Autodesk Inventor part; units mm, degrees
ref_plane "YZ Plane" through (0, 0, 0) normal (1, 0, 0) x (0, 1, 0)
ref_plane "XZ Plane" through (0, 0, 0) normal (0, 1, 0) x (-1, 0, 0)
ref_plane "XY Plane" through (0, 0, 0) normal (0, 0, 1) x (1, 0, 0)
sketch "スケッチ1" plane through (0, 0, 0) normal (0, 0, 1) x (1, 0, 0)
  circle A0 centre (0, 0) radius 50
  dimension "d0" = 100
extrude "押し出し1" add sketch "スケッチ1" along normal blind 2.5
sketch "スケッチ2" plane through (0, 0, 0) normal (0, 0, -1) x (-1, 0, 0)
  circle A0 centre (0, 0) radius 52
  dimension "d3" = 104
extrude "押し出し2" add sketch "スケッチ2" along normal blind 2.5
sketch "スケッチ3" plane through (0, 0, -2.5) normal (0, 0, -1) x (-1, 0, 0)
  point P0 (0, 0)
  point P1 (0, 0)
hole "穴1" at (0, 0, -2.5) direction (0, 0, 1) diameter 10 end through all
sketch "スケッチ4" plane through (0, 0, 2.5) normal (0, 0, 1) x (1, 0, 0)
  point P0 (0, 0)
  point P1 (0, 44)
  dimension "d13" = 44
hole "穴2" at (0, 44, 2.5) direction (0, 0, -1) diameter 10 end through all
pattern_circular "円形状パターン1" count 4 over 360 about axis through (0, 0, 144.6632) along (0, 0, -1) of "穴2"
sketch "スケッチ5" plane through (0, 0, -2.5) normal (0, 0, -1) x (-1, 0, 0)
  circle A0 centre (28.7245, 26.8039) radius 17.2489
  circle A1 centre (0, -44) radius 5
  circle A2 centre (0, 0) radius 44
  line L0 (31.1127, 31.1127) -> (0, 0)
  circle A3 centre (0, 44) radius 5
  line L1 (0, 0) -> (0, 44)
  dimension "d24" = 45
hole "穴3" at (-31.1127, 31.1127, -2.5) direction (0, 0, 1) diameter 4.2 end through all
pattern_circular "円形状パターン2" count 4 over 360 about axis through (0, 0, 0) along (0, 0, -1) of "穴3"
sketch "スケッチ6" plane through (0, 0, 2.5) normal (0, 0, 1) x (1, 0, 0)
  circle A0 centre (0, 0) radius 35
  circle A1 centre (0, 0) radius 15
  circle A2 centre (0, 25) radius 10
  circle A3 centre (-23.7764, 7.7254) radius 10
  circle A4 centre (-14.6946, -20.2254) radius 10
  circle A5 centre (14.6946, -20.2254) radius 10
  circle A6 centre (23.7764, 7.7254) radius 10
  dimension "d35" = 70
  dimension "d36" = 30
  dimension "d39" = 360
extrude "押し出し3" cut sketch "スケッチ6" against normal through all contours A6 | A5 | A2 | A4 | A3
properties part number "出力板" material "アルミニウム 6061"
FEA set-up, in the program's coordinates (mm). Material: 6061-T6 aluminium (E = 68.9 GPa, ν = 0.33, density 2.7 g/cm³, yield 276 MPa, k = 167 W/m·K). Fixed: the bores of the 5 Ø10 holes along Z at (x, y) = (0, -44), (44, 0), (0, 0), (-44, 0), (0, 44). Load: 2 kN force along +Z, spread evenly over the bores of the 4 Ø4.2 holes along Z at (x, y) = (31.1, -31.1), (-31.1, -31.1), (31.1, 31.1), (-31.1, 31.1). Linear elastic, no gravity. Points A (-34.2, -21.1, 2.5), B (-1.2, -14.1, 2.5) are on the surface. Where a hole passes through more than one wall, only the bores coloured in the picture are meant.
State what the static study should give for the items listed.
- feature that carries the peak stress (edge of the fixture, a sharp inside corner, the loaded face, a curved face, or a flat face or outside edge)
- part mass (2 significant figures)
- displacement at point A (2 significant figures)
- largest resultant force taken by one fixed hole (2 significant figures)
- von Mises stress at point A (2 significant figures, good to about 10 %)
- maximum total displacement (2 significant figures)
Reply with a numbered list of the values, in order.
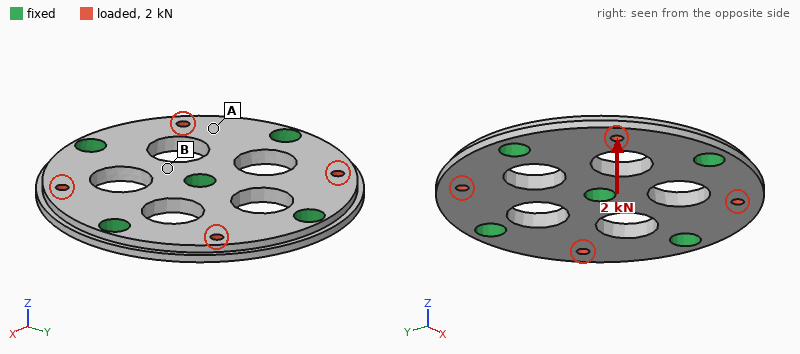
1. the loaded face
2. 83 g
3. 34 µm
4. 510 N
5. 20 MPa
6. 80 µm
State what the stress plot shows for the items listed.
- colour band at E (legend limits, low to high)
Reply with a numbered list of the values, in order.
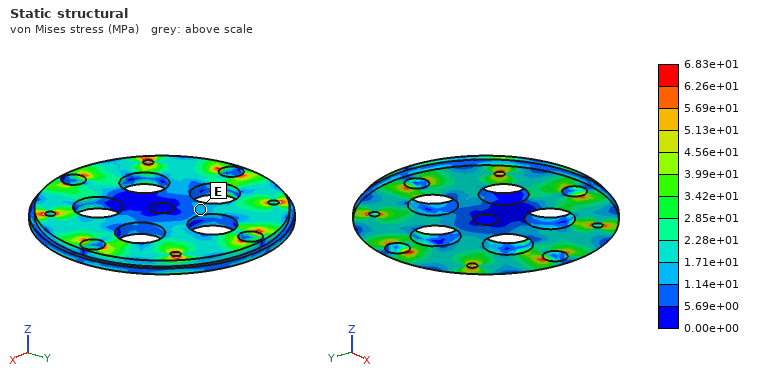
1. 1.14e+01 to 1.71e+01 MPa
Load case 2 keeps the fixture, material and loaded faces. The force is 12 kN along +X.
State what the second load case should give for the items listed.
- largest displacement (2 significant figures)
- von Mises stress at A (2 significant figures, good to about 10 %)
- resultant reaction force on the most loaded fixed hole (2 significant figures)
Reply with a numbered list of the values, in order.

1. 19 µm
2. 18 MPa
3. 4.0 kN
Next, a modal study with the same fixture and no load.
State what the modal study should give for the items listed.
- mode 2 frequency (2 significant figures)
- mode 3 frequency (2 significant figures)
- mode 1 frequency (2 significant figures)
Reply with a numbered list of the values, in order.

1. 6500 Hz
2. 6600 Hz
3. 6400 Hz
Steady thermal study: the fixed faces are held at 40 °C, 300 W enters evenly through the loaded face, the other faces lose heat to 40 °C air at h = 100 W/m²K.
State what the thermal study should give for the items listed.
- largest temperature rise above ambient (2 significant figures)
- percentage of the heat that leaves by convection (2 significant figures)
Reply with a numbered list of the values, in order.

1. 73 K
2. 13 %
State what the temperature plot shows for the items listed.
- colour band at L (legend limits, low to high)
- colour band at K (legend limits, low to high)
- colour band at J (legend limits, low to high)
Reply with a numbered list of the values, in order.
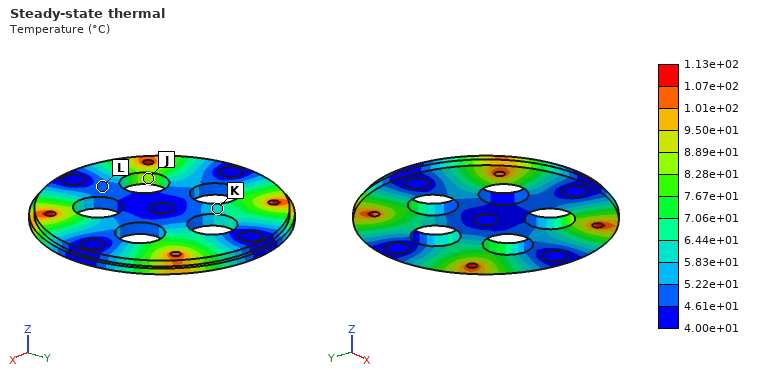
1. 4.61e+01 to 5.22e+01 °C
2. 5.83e+01 to 6.44e+01 °C
3. 8.28e+01 to 8.89e+01 °C
